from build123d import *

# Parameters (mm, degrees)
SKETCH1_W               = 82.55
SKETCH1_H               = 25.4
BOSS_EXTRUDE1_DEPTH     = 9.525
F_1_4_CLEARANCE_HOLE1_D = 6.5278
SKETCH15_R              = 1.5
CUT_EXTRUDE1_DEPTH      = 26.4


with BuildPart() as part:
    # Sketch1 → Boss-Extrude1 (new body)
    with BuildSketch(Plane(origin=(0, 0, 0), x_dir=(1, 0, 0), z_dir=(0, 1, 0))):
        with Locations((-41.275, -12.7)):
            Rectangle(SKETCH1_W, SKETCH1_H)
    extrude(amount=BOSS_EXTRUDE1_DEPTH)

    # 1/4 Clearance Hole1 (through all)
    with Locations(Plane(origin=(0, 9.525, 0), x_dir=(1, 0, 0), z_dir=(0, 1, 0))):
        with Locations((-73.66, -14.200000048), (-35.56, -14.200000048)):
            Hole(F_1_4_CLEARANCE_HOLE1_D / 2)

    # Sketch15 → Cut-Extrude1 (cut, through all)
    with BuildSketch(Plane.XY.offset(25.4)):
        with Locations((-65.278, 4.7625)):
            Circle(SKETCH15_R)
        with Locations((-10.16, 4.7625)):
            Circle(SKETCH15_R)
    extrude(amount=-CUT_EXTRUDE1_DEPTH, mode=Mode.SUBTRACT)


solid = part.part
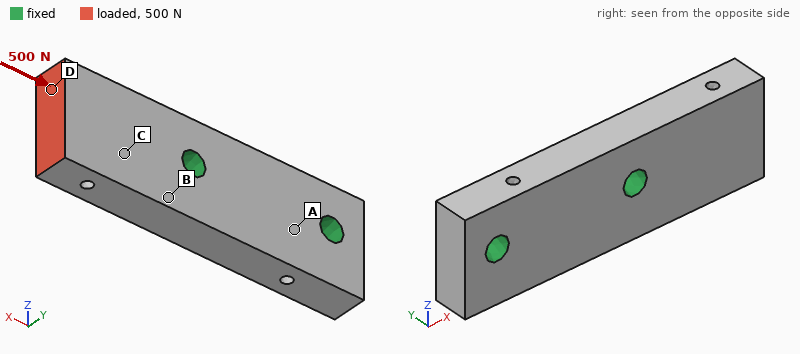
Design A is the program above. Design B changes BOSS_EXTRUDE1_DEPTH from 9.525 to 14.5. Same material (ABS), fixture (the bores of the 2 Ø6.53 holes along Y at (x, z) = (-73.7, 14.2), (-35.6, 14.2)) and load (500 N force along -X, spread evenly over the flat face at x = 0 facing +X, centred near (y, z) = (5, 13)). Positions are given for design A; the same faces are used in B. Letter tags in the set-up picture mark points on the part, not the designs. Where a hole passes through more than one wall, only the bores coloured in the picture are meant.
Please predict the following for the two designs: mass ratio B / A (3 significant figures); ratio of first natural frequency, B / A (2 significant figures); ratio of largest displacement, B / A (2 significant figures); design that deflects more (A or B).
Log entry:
1.53
1.4
0.66
A
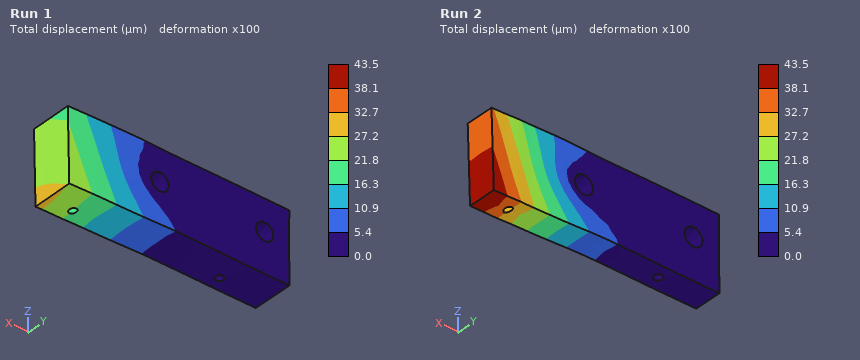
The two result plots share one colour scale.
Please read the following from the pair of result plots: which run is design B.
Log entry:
Run 1
